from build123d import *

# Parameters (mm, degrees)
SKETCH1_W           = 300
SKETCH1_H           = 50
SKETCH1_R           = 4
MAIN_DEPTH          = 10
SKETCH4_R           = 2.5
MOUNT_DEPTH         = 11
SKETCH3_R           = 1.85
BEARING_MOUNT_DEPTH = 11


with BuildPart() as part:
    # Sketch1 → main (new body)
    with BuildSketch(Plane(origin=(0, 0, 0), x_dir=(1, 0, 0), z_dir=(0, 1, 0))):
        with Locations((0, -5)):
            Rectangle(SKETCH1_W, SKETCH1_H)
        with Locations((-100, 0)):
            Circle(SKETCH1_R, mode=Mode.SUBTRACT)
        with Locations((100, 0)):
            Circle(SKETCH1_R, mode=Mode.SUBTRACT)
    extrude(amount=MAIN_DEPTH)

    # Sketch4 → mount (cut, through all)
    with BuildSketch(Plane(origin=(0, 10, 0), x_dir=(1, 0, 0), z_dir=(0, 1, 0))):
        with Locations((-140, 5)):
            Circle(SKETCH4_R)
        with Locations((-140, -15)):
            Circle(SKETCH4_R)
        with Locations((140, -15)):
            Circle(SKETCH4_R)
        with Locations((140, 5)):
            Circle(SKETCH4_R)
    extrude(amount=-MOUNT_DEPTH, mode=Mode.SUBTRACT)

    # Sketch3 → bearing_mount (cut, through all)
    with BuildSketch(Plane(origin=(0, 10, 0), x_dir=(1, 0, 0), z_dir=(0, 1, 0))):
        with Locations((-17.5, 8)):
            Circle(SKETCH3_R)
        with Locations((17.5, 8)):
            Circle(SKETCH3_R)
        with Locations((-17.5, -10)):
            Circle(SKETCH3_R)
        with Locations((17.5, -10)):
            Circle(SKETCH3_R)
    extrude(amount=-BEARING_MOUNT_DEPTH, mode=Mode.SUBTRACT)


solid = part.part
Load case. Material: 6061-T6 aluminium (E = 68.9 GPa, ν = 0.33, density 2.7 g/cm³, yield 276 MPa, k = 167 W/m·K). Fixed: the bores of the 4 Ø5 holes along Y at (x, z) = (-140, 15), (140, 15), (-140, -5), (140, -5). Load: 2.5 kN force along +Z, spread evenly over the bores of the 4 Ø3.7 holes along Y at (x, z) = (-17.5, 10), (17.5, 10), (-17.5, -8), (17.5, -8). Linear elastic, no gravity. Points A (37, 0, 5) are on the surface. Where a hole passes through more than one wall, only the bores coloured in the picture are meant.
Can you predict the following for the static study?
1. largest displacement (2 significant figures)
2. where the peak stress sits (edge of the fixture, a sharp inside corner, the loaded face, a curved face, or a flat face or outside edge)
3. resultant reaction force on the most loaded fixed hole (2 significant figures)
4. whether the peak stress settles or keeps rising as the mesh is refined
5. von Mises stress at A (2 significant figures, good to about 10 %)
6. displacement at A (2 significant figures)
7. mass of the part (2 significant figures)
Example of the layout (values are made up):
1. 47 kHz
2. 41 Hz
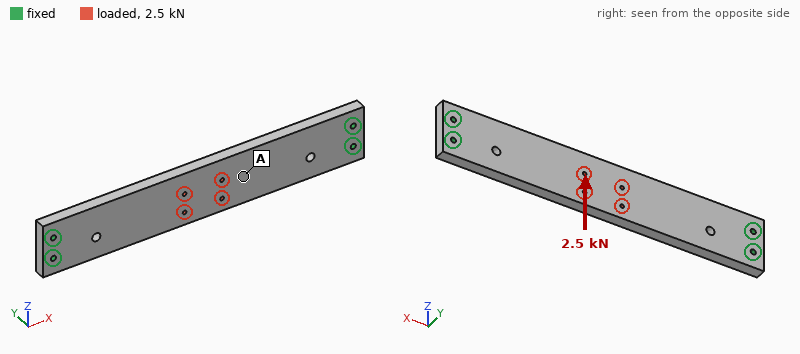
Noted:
1. 69 µm
2. edge of the fixture
3. 3.2 kN
4. keeps rising
5. 6.3 MPa
6. 59 µm
7. 400 g
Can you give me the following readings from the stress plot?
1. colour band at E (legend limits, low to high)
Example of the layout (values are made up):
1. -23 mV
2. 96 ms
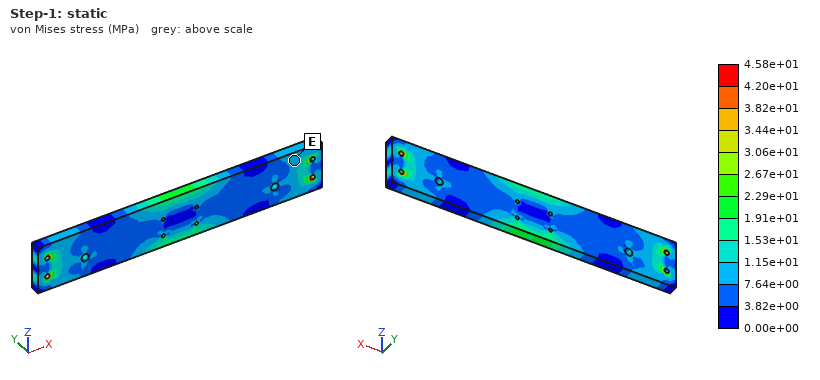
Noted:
1. 7.64e+00 to 1.15e+01 MPa
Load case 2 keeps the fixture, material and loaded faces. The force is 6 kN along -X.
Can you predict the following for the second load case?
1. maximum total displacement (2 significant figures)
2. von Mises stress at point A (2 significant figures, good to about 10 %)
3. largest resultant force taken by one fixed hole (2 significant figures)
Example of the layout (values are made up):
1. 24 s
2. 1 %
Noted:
1. 13 µm
2. 6.9 MPa
3. 1.6 kN
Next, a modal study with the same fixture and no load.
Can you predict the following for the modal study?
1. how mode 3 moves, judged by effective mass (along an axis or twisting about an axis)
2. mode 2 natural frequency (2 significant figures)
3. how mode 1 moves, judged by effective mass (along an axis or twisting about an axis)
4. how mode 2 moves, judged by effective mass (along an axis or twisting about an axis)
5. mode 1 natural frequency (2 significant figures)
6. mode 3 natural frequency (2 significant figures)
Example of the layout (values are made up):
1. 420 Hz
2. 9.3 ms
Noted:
1. twisting about X
2. 1800 Hz
3. along Y
4. twisting about Z
5. 650 Hz
6. 2100 Hz
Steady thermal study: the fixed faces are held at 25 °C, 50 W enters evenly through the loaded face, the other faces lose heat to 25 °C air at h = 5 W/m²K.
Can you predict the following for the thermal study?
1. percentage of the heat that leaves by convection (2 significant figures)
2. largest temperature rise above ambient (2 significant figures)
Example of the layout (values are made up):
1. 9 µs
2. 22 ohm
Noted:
1. 6.9 %
2. 38 K
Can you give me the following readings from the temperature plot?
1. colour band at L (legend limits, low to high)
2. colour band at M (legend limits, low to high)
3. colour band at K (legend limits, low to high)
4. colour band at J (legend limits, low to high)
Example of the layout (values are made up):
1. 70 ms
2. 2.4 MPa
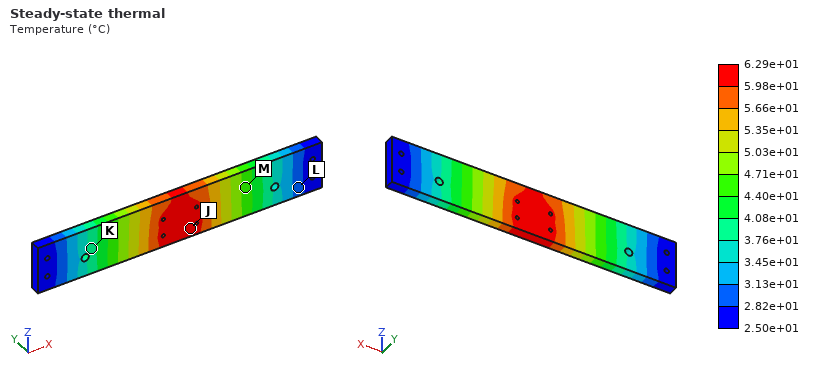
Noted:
1. 2.82e+01 to 3.13e+01 °C
2. 4.40e+01 to 4.71e+01 °C
3. 3.76e+01 to 4.08e+01 °C
4. 5.98e+01 to 6.29e+01 °C
